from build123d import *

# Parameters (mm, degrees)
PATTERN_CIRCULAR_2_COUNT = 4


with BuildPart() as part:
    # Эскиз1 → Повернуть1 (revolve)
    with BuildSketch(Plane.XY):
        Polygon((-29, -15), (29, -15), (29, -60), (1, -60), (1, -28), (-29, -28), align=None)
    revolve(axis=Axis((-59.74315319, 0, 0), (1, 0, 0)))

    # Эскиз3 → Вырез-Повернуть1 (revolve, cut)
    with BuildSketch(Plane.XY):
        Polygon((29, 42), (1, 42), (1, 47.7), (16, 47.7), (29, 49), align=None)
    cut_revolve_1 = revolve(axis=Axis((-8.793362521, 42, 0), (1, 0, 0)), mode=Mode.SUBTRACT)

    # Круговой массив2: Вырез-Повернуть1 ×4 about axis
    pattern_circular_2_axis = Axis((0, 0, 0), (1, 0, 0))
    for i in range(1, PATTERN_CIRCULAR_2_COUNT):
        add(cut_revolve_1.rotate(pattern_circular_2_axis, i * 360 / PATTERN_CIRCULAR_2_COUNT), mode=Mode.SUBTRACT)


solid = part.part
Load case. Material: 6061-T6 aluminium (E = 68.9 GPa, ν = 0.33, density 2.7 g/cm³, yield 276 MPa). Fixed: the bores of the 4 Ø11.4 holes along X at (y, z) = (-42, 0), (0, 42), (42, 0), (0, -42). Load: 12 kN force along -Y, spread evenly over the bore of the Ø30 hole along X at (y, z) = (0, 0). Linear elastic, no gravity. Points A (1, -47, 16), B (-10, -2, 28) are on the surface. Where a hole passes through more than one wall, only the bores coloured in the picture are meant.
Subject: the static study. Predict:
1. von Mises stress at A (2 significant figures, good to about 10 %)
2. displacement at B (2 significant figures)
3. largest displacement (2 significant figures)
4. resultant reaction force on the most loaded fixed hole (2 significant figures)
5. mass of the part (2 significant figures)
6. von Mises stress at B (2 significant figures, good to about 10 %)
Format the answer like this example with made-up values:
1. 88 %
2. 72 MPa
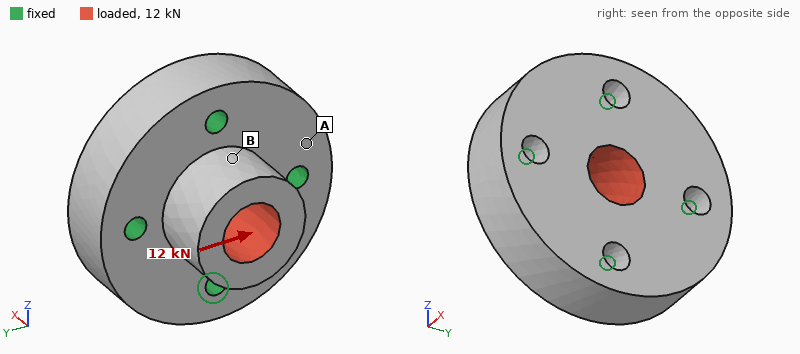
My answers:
1. 2.2 MPa
2. 4.3 µm
3. 9.2 µm
4. 3.8 kN
5. 910 g
6. 4.6 MPa
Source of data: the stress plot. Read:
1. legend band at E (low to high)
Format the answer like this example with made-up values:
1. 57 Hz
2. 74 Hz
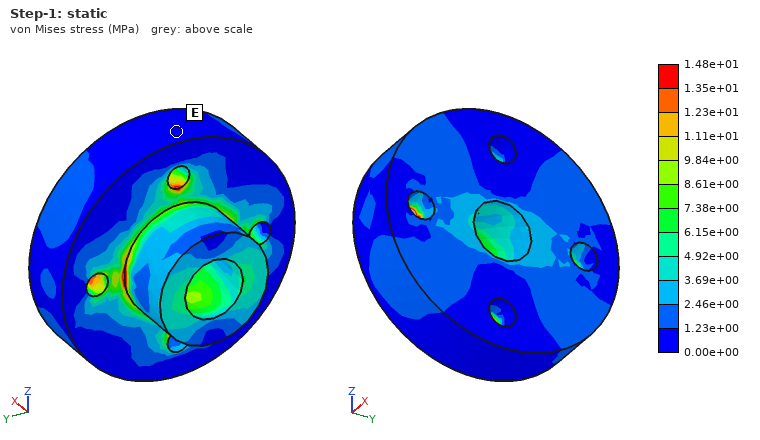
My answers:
1. 0.00e+00 to 1.23e+00 MPa
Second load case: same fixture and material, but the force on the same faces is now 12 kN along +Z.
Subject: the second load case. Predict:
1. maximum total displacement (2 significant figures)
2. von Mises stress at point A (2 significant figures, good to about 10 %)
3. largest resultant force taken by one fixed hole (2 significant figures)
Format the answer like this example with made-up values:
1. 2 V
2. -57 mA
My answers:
1. 9.2 µm
2. 1.7 MPa
3. 3.8 kN
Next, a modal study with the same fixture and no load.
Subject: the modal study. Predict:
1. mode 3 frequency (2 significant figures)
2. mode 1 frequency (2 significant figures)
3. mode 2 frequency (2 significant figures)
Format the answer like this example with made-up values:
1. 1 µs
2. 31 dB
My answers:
1. 12 kHz
2. 12 kHz
3. 12 kHz
